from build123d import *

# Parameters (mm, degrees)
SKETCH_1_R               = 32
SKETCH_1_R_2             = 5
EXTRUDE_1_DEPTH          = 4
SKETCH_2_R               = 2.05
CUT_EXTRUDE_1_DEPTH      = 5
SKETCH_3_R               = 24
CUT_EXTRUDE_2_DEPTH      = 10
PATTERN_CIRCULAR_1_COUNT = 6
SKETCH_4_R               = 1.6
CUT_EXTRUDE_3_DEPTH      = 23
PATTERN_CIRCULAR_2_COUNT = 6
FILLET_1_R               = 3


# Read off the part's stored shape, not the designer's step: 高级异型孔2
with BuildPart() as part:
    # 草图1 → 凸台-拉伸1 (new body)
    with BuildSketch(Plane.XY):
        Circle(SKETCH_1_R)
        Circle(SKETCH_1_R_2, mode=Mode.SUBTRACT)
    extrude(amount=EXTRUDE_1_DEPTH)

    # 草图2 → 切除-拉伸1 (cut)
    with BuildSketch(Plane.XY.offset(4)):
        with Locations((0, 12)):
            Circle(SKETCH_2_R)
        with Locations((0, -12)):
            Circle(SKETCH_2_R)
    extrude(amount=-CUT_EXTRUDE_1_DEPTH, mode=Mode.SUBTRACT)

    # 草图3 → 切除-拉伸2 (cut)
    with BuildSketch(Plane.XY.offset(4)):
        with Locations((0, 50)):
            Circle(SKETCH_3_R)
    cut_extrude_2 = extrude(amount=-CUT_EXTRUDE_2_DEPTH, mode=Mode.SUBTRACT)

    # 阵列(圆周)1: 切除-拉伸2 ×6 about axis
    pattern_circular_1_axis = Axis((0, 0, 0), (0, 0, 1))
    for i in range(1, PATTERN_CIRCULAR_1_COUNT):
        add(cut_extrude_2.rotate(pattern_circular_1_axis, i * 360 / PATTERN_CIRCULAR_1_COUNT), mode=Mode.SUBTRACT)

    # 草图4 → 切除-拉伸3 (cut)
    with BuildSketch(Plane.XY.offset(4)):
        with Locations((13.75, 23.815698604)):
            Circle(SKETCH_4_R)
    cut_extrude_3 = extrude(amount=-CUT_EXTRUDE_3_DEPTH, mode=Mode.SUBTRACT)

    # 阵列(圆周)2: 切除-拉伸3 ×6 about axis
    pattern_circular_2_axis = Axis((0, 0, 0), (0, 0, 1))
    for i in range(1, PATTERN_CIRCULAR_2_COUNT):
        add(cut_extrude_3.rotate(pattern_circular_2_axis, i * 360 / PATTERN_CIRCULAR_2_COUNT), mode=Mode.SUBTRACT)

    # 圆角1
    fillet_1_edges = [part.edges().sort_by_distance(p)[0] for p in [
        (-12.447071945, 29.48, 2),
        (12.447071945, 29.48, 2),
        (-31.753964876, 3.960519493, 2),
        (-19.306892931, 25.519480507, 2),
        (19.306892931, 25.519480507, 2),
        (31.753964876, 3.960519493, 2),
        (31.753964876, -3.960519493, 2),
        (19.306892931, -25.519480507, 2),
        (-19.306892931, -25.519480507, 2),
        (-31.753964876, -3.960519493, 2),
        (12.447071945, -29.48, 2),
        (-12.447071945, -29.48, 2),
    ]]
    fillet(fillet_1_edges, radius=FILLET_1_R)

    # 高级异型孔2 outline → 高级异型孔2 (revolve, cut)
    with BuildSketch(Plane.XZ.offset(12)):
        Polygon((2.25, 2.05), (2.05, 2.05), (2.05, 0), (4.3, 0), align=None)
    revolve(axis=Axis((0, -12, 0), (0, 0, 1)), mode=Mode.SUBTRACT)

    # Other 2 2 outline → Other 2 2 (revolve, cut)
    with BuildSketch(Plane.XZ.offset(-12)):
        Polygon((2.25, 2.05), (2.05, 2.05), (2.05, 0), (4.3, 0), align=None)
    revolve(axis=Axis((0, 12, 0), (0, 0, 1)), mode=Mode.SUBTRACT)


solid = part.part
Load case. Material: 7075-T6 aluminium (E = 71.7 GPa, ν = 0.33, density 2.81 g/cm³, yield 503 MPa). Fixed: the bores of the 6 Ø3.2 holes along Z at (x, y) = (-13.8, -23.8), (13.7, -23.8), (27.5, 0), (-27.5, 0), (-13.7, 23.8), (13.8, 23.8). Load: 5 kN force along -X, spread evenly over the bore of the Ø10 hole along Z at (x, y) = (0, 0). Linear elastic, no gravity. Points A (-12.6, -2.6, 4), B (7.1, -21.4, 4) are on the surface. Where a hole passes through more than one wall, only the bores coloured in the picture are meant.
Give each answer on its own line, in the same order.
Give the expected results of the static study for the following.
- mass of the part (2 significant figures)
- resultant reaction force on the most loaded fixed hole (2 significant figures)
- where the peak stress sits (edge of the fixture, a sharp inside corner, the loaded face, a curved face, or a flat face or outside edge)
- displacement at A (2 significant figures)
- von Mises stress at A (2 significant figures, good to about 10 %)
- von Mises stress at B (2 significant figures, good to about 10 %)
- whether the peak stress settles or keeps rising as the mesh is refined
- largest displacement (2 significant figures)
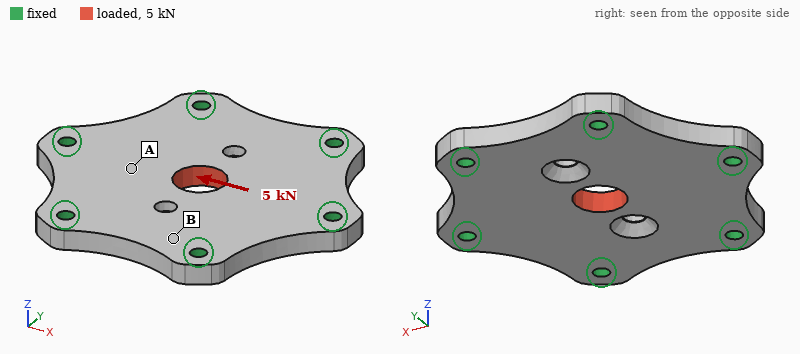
27 g
1.5 kN
edge of the fixture
6.7 µm
29 MPa
11 MPa
keeps rising
11 µm
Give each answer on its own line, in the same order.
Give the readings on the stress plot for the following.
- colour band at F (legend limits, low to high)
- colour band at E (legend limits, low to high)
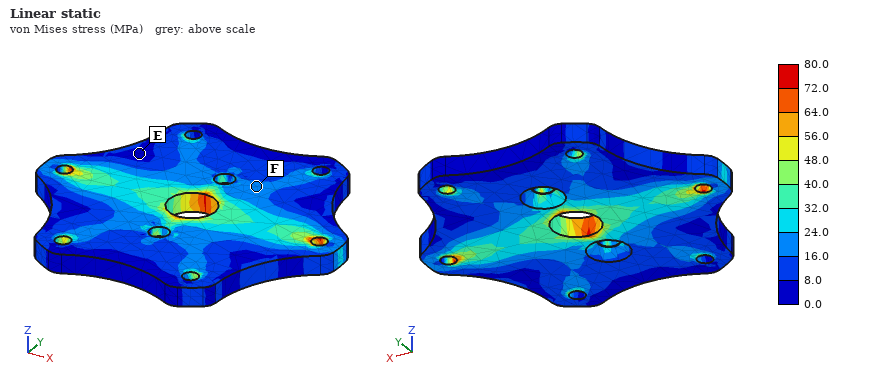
16.0 to 24.0 MPa
0.0 to 8.0 MPa
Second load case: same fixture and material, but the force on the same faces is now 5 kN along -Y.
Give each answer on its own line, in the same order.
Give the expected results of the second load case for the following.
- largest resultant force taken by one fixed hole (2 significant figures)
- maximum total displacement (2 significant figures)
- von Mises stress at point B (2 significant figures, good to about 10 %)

1.2 kN
13 µm
20 MPa
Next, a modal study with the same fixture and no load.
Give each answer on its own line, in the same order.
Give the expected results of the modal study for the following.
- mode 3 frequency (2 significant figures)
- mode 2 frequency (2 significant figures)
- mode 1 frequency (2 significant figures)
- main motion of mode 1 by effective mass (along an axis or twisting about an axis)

20 kHz
20 kHz
10 kHz
along Z
